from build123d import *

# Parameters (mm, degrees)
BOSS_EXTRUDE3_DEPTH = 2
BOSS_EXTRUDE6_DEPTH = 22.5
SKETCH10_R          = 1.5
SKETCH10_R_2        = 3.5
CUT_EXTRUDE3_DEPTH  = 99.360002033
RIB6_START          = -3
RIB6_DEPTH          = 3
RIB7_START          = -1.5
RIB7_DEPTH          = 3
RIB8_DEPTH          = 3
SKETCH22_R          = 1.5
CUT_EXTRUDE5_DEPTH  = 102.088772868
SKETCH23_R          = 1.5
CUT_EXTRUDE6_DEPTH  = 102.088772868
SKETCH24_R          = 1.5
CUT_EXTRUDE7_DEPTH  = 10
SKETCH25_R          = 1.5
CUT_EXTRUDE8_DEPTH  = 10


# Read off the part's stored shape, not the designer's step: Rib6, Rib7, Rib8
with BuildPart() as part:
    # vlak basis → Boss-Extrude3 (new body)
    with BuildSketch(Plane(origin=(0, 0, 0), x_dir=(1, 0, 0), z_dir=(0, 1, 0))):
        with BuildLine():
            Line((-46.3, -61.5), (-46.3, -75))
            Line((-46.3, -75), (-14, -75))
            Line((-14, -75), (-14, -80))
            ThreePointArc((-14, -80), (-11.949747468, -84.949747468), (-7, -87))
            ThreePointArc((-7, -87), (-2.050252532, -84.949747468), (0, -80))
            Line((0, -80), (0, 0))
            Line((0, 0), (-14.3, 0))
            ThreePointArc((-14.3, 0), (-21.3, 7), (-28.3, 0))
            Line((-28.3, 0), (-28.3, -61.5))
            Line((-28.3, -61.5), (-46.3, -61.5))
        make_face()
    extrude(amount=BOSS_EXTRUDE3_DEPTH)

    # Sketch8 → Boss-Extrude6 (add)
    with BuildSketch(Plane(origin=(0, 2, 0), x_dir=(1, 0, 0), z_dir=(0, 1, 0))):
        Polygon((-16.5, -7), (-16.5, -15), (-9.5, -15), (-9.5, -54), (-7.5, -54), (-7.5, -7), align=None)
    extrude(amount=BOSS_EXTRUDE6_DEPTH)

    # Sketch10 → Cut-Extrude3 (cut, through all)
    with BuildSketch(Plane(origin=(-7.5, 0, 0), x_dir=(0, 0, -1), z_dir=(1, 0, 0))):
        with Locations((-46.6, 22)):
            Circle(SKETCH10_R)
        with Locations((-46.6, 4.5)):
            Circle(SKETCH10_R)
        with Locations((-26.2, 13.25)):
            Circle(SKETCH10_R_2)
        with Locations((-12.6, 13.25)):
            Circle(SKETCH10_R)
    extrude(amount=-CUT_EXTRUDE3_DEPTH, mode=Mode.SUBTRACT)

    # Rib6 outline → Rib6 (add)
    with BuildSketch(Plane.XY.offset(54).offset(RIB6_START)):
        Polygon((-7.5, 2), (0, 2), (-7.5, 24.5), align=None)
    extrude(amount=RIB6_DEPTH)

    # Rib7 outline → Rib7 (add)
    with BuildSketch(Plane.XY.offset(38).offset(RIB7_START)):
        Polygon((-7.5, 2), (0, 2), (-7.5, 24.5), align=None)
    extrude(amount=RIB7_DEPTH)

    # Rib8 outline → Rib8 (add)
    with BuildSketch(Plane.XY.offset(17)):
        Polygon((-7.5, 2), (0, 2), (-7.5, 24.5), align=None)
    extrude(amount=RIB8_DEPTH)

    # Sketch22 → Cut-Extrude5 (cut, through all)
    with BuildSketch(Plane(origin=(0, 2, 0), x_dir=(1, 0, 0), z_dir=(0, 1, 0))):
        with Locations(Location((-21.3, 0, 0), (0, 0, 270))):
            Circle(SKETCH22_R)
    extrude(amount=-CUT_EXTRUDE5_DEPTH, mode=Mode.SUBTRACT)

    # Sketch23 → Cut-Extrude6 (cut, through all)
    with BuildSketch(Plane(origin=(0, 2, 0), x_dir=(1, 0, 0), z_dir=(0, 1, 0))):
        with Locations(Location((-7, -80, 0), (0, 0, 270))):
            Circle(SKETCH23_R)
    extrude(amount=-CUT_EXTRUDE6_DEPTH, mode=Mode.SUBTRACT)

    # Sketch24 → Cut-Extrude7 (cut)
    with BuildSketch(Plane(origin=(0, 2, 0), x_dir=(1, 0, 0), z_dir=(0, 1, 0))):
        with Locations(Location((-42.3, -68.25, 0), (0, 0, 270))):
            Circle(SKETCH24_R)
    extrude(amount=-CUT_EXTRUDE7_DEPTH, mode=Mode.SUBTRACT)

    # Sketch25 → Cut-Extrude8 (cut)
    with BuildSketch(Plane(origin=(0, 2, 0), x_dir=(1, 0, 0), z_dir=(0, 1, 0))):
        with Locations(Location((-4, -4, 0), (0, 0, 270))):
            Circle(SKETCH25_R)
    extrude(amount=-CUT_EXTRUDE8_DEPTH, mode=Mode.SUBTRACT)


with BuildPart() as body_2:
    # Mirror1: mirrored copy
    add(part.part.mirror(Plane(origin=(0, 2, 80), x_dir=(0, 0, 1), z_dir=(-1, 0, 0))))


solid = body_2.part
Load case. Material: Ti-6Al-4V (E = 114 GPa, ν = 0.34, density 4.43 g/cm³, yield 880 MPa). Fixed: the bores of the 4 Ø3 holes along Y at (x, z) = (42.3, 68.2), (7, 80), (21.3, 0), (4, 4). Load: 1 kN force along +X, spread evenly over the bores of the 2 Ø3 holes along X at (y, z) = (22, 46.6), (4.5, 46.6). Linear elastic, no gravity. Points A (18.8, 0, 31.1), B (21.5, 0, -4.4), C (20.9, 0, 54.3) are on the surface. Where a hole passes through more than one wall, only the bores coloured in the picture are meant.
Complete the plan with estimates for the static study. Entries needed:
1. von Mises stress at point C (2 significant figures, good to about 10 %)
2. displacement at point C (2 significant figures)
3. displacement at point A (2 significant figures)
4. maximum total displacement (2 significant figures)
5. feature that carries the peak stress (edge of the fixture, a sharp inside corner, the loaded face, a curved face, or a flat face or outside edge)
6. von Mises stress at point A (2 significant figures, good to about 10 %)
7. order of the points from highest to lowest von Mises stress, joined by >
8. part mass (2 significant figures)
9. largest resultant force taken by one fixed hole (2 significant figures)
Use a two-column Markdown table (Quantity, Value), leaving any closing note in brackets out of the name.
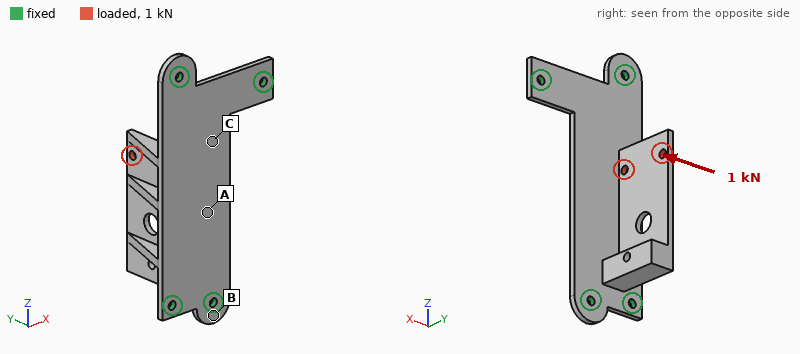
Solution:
| Quantity | Value |
|---|---|
| von Mises stress at point C | 83 MPa |
| displacement at point C | 0.12 mm |
| displacement at point A | 0.11 mm |
| maximum total displacement | 0.71 mm |
| feature that carries the peak stress | the loaded face |
| von Mises stress at point A | 48 MPa |
| order of the points from highest to lowest von Mises stress, joined by > | C > A > B |
| part mass | 40 g |
| largest resultant force taken by one fixed hole | 760 N |
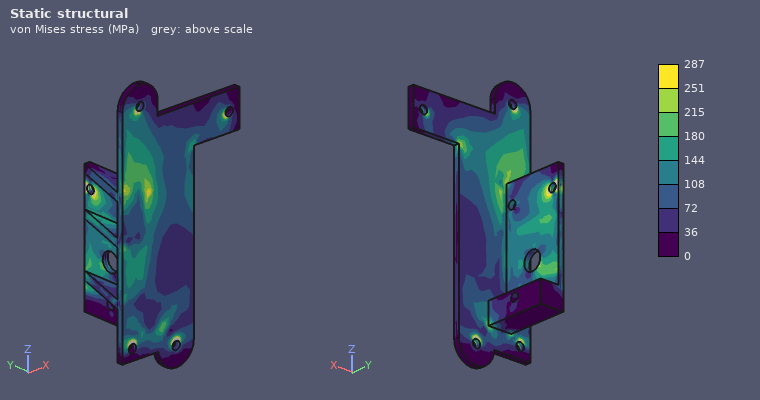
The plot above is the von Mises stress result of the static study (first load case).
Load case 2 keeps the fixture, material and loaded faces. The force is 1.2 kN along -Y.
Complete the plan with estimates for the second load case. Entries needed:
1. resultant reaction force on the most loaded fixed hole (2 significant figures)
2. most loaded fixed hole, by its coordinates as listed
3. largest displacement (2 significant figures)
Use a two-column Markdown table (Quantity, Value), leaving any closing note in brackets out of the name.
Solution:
| Quantity | Value |
|---|---|
| resultant reaction force on the most loaded fixed hole | 650 N |
| most loaded fixed hole, by its coordinates as listed | (7, 80) |
| largest displacement | 0.70 mm |
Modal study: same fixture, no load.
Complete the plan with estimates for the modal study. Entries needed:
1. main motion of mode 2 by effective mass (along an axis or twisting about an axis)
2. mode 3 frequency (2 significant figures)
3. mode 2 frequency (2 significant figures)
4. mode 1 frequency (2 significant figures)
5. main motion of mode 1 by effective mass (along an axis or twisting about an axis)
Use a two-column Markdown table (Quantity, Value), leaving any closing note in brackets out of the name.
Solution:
| Quantity | Value |
|---|---|
| main motion of mode 2 by effective mass | along X |
| mode 3 frequency | 4900 Hz |
| mode 2 frequency | 2600 Hz |
| mode 1 frequency | 1900 Hz |
| main motion of mode 1 by effective mass | along Y |
